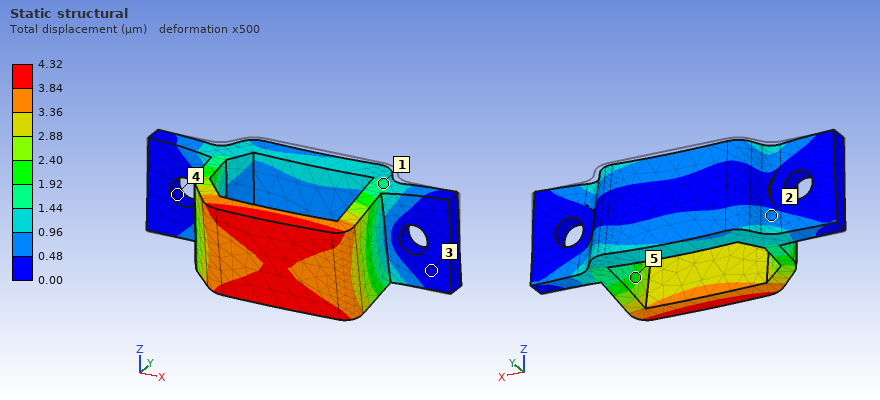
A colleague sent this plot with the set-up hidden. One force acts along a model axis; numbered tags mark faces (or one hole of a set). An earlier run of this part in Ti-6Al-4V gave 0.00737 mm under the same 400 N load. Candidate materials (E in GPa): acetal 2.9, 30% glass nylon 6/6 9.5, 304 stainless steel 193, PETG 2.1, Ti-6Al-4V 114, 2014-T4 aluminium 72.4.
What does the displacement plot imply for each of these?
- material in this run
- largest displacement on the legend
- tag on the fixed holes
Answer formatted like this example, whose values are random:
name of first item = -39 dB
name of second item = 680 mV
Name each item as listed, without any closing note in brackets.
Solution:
material in this run = 304 stainless steel
largest displacement on the legend = 4.32 µm
tag on the fixed holes = 4
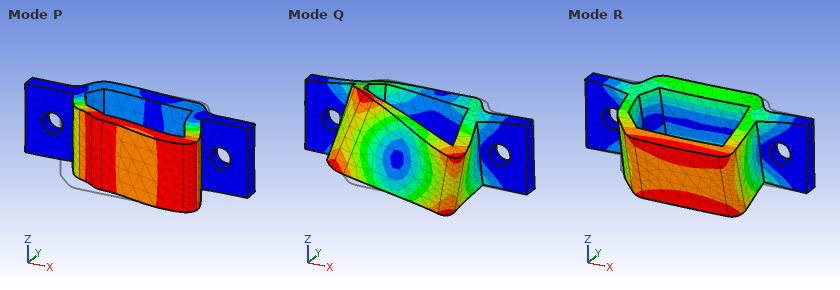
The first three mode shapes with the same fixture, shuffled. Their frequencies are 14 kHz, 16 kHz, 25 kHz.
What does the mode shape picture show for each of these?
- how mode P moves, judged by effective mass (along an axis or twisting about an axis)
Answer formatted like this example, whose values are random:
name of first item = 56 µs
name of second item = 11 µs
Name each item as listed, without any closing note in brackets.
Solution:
how mode P moves, judged by effective mass = along X
